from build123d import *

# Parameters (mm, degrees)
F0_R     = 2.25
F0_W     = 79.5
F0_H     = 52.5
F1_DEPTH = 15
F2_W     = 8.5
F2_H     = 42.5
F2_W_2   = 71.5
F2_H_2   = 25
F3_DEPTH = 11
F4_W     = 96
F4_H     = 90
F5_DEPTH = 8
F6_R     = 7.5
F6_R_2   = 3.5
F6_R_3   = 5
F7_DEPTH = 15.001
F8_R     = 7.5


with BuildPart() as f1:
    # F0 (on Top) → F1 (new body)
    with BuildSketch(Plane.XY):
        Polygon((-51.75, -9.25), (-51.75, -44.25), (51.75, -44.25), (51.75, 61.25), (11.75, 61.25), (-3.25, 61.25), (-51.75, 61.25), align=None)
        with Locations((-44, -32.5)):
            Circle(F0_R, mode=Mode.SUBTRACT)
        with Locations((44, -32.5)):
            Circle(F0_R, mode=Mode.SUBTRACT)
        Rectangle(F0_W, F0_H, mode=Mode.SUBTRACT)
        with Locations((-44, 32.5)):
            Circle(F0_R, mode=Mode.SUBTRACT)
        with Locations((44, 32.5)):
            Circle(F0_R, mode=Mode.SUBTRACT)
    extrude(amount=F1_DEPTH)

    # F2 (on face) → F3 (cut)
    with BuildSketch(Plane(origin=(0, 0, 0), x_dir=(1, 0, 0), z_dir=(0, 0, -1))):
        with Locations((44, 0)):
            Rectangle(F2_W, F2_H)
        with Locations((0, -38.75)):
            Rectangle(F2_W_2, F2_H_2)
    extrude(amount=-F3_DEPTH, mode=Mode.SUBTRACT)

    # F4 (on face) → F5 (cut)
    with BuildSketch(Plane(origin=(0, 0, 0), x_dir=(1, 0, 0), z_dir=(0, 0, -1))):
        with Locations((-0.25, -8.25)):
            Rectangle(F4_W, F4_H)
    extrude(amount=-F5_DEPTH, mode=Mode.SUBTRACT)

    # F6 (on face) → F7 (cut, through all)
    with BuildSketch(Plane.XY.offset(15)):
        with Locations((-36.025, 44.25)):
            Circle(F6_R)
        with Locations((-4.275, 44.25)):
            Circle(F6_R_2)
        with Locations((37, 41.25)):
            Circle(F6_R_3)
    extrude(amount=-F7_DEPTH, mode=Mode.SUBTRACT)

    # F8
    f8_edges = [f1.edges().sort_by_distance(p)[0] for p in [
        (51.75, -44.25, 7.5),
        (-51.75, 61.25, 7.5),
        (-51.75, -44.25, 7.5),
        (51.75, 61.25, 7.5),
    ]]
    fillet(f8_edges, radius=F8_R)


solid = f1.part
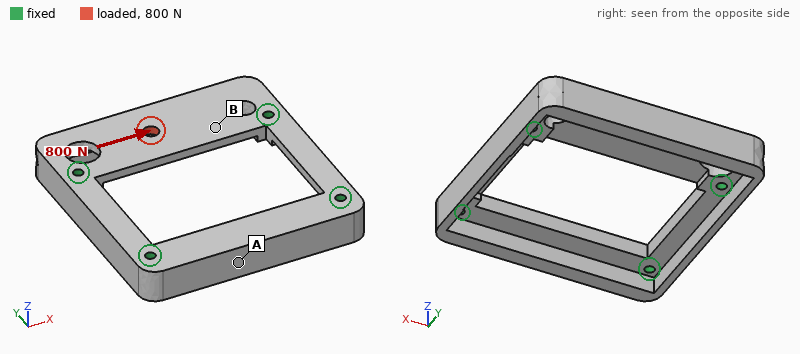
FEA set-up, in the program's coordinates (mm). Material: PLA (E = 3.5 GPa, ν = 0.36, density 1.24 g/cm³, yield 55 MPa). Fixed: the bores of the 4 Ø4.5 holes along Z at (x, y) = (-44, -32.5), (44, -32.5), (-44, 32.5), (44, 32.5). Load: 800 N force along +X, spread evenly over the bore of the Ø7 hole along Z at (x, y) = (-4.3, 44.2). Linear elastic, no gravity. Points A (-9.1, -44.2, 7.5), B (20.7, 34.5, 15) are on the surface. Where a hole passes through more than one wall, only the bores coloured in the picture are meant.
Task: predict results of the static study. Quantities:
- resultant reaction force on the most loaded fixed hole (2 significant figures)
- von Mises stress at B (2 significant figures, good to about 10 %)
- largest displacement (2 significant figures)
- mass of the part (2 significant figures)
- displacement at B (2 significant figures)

410 N
4.7 MPa
84 µm
70 g
40 µm
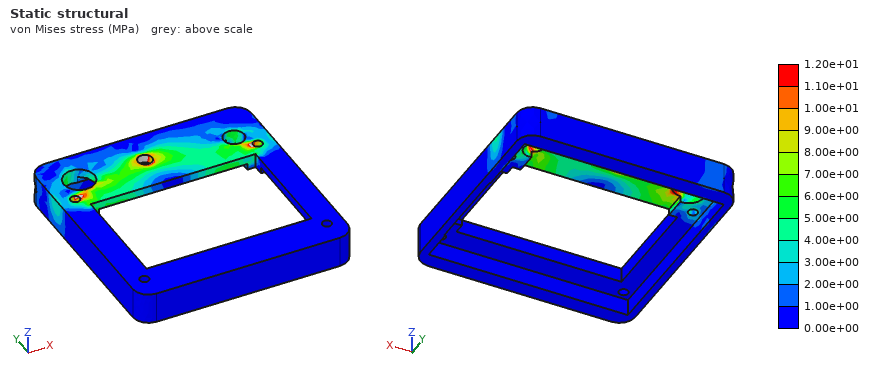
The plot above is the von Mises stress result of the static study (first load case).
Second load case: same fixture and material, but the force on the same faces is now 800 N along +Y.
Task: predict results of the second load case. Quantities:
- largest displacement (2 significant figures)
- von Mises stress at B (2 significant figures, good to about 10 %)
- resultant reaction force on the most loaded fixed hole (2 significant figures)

0.27 mm
4.9 MPa
540 N
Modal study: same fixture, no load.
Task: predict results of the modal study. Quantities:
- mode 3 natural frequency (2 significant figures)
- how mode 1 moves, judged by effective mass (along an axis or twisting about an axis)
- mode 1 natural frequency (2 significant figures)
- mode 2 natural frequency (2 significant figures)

1800 Hz
along Z
960 Hz
1600 Hz
